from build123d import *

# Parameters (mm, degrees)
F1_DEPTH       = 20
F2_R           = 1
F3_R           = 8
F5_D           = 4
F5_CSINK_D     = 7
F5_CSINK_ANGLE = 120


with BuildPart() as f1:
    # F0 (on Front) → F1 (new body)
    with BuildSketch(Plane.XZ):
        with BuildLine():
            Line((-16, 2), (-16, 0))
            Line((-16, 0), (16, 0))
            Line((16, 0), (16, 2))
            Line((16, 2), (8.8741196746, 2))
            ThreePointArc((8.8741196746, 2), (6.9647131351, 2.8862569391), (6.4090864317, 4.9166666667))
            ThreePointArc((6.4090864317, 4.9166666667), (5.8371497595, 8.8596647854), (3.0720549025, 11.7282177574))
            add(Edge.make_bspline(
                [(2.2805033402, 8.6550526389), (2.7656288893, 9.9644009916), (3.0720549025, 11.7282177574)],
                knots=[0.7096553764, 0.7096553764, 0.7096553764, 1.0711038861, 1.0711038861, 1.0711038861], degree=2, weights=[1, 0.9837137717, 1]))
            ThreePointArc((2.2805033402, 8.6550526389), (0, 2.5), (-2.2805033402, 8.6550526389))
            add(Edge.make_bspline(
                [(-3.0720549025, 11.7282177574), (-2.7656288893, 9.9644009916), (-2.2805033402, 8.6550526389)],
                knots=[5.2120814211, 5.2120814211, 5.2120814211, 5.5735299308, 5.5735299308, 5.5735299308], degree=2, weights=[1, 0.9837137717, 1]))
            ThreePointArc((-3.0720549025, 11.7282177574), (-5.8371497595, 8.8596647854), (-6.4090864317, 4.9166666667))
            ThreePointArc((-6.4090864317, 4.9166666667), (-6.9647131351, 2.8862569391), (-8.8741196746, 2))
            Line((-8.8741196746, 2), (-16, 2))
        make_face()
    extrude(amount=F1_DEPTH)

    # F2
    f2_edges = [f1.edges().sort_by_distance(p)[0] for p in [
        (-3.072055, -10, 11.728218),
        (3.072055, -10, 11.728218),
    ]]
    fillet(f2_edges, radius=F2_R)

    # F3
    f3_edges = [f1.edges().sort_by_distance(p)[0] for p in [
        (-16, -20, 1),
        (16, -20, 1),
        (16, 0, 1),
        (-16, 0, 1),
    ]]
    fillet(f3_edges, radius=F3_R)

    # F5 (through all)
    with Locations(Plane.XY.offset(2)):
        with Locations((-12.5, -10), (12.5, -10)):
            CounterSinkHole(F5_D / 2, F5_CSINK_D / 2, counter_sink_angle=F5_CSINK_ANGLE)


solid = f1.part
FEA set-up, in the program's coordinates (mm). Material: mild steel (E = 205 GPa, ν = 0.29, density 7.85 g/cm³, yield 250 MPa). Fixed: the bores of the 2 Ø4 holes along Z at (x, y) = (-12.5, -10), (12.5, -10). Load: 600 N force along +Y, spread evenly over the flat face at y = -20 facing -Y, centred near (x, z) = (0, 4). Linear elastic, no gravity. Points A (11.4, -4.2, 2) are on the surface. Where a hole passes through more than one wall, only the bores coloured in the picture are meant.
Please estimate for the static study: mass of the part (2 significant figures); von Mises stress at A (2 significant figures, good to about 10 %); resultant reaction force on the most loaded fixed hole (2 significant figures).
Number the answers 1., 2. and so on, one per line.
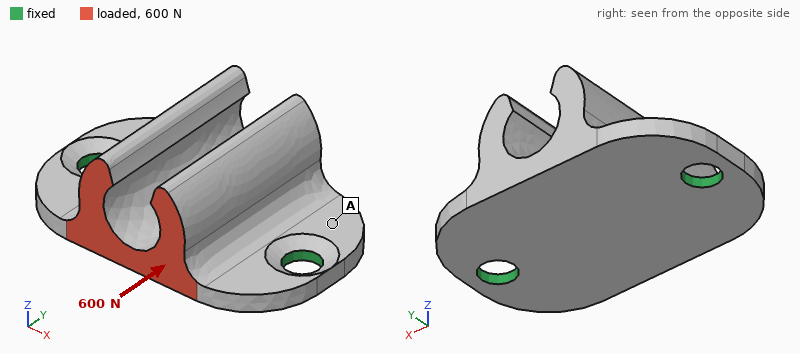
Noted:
1. 19 g
2. 21 MPa
3. 300 N
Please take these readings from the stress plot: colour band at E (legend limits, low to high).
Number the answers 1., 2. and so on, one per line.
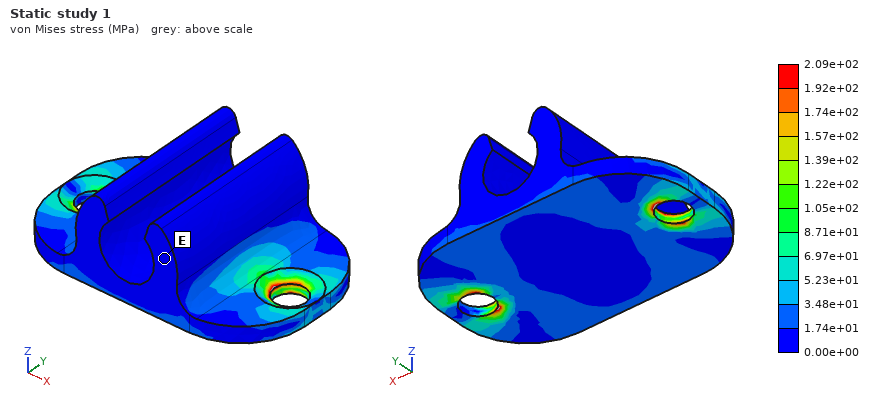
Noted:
1. 0.00e+00 to 1.74e+01 MPa
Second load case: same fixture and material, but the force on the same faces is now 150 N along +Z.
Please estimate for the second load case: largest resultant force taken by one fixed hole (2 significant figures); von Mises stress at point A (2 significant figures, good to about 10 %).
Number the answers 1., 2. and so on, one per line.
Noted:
1. 120 N
2. 12 MPa
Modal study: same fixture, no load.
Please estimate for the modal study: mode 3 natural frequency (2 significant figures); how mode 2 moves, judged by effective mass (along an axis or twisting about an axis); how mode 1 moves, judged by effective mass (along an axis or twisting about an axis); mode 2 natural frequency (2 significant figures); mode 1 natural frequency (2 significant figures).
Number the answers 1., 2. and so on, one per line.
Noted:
1. 22 kHz
2. along Z
3. along Y
4. 11 kHz
5. 6300 Hz
